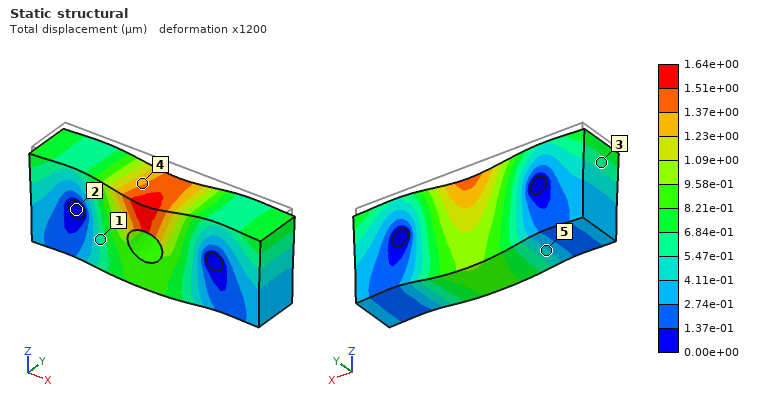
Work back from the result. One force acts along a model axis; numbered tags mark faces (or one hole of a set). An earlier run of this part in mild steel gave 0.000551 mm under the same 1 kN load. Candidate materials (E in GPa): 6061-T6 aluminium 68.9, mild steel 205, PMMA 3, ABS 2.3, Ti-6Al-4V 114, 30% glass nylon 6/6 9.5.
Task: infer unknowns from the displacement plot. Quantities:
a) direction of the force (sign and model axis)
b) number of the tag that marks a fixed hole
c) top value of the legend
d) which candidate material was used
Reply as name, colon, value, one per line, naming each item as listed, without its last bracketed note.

direction of the force: -Z
number of the tag that marks a fixed hole: 2
top value of the legend: 1.64e+00 µm
which candidate material was used: 6061-T6 aluminium
